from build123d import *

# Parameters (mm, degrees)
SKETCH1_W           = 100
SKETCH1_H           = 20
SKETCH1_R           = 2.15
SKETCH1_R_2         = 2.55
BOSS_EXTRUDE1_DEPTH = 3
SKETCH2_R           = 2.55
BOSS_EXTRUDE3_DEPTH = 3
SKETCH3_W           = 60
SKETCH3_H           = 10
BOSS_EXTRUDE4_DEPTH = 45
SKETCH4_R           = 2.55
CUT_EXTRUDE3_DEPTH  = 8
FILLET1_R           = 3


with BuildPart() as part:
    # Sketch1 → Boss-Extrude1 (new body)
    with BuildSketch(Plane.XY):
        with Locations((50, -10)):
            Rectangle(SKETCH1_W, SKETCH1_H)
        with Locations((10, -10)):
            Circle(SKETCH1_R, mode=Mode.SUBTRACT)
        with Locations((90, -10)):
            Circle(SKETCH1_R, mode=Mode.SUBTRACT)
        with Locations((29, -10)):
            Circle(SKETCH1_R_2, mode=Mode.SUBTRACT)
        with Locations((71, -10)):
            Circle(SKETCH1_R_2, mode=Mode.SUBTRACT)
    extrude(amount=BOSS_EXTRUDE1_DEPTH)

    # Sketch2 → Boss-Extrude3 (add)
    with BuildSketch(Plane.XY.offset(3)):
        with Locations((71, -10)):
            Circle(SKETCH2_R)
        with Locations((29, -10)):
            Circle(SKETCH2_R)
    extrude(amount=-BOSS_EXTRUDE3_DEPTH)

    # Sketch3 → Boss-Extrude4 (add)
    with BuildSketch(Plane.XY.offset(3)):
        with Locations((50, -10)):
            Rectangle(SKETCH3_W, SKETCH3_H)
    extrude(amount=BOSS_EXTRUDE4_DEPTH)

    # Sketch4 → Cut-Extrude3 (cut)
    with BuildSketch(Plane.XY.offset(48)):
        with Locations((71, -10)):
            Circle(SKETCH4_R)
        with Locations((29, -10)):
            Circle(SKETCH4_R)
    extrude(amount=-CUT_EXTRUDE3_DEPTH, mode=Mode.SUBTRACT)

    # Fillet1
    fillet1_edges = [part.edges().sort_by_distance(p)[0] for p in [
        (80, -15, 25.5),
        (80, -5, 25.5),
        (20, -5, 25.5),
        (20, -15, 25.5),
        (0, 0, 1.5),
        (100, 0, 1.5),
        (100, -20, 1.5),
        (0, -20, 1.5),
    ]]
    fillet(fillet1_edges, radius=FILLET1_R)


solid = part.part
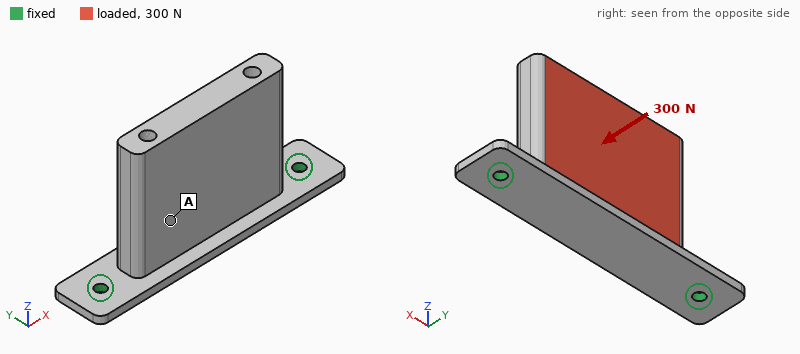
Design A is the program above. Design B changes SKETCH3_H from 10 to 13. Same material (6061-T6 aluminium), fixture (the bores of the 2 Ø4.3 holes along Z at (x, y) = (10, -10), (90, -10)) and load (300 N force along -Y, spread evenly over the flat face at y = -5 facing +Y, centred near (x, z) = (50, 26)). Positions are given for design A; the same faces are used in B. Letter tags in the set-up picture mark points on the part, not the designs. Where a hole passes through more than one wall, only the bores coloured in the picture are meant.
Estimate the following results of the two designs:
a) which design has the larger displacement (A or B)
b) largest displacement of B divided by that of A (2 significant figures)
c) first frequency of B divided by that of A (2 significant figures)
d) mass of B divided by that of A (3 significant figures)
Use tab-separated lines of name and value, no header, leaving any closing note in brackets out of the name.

which design has the larger displacement	A
largest displacement of B divided by that of A	0.87
first frequency of B divided by that of A	0.93
mass of B divided by that of A	1.25
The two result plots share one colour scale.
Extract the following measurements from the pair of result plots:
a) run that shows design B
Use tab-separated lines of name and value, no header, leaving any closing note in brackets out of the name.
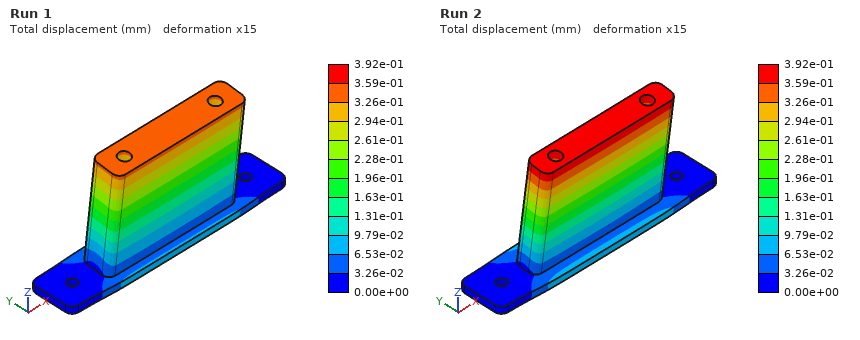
run that shows design B	Run 1
